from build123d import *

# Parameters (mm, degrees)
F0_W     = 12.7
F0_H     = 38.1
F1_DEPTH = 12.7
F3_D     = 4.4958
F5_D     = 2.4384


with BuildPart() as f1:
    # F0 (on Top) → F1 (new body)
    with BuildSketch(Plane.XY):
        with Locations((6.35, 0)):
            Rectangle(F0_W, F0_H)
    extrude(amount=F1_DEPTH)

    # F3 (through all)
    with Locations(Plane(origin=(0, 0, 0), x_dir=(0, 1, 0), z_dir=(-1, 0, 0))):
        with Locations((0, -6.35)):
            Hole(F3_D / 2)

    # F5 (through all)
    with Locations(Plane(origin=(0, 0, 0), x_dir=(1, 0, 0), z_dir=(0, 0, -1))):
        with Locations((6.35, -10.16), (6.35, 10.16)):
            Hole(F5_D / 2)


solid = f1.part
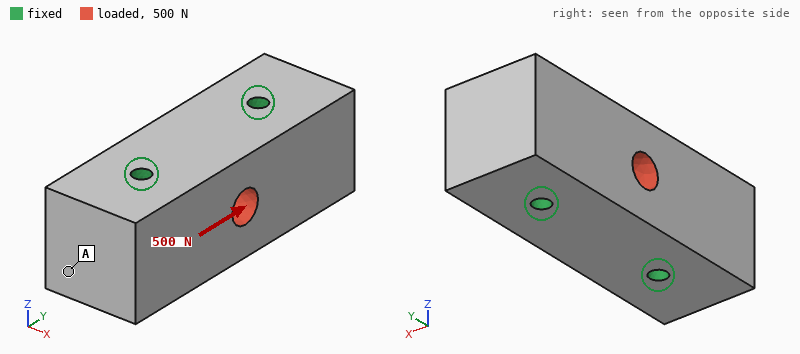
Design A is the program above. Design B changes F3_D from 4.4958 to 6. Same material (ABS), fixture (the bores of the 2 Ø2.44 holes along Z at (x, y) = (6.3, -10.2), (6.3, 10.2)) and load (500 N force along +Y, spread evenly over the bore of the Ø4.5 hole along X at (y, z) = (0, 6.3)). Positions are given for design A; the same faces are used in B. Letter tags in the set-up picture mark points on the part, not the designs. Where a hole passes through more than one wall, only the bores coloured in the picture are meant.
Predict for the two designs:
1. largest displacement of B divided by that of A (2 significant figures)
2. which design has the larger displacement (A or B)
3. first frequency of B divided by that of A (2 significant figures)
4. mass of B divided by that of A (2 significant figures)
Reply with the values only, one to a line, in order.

0.91
A
0.97
0.97
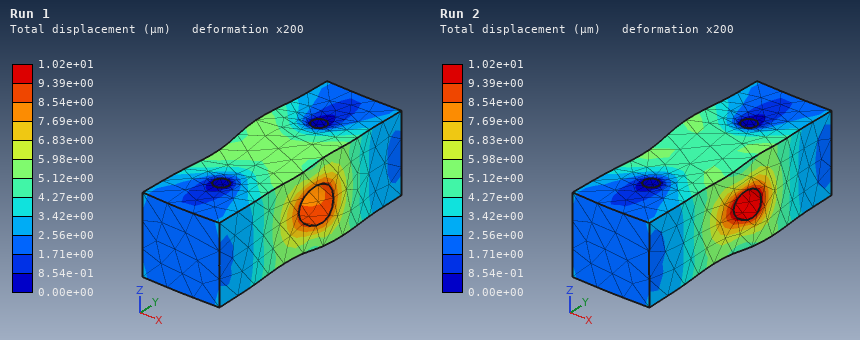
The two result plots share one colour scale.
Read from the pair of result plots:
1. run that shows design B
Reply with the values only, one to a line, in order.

Run 1
